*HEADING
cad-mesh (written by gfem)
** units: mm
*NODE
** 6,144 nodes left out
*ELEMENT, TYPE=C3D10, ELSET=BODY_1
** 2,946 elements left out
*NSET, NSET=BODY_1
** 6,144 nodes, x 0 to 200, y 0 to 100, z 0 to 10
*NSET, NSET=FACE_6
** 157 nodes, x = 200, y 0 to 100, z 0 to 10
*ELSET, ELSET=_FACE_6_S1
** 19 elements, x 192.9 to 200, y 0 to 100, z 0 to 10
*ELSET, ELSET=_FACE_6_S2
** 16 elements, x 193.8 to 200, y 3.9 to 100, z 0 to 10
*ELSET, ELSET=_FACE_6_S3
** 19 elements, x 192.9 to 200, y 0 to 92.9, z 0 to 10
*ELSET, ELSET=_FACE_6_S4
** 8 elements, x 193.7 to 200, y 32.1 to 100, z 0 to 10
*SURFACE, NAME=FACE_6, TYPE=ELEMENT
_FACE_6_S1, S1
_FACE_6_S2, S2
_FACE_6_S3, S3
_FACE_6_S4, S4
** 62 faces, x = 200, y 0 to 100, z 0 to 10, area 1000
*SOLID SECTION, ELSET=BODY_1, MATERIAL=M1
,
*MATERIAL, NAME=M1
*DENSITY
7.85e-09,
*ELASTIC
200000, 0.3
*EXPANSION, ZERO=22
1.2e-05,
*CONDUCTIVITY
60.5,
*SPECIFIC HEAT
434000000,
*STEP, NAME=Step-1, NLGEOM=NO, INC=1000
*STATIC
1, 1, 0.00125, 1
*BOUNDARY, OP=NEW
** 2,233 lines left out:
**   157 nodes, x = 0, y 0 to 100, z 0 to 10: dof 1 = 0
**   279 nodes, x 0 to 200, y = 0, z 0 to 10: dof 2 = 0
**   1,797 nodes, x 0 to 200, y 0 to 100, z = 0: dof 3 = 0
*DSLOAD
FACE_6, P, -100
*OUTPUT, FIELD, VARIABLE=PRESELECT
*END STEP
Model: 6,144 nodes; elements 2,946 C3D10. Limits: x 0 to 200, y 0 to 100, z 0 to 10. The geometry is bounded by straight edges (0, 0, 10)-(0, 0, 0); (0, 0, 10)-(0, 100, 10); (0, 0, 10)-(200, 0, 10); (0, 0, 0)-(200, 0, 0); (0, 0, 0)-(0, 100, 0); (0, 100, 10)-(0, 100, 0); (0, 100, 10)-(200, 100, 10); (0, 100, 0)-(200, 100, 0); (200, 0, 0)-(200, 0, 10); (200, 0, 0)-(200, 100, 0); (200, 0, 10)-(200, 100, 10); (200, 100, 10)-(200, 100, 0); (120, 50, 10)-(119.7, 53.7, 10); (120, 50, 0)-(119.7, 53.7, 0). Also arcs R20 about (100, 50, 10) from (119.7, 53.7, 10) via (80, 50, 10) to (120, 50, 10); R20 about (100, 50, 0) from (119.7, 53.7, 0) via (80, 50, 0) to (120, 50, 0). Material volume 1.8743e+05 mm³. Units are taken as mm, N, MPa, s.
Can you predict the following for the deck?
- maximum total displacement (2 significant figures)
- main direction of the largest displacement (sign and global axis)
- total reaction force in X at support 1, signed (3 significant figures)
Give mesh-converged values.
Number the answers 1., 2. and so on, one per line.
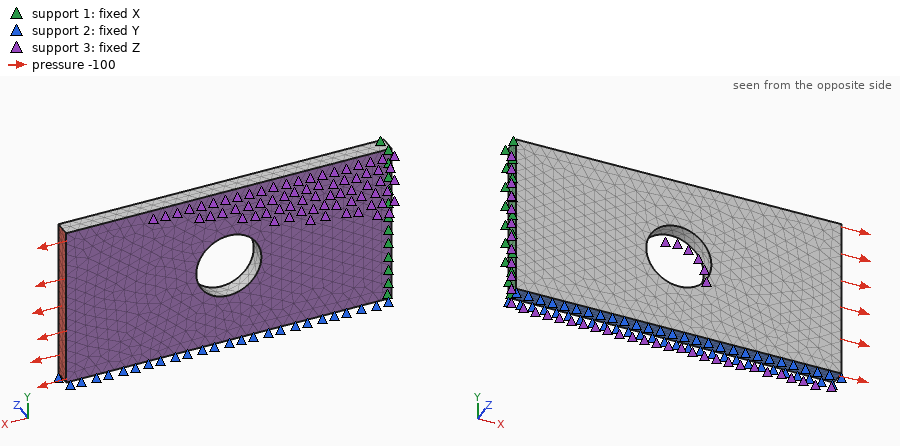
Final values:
1. 0.12 mm
2. +X
3. -100000 N
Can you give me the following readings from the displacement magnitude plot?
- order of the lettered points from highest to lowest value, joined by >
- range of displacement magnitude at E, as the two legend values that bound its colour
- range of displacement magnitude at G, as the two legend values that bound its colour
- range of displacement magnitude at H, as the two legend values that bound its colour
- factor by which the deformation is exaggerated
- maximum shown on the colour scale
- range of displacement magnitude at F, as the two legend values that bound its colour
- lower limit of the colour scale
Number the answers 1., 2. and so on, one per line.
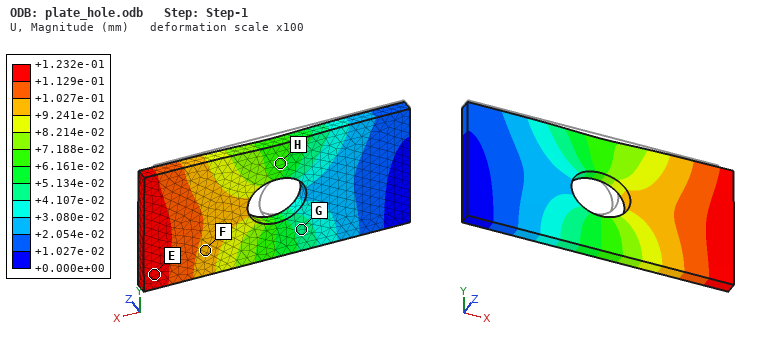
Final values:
1. E > F > H > G
2. +1.129e-01 to +1.232e-01 mm
3. +4.107e-02 to +5.134e-02 mm
4. +6.161e-02 to +7.188e-02 mm
5. 100
6. +1.232e-01 mm
7. +9.241e-02 to +1.027e-01 mm
8. +0.000e+00 mm
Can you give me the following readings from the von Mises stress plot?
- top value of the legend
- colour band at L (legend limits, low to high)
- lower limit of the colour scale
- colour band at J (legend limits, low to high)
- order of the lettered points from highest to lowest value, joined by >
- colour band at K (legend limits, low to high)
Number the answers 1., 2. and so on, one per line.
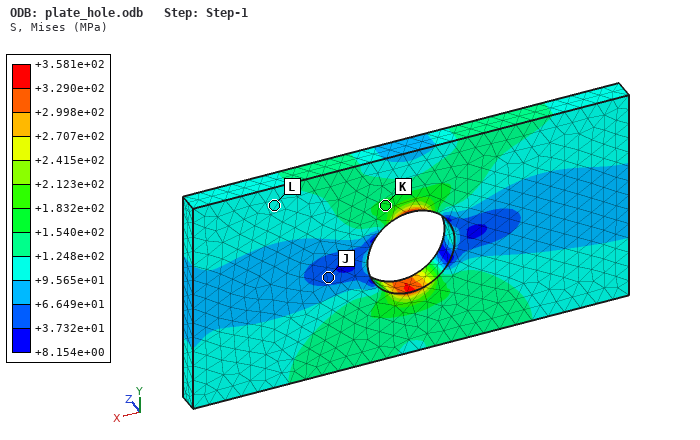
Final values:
1. +3.581e+02 MPa
2. +9.565e+01 to +1.248e+02 MPa
3. +8.154e+00 MPa
4. +3.732e+01 to +6.649e+01 MPa
5. K > L > J
6. +1.540e+02 to +1.832e+02 MPa
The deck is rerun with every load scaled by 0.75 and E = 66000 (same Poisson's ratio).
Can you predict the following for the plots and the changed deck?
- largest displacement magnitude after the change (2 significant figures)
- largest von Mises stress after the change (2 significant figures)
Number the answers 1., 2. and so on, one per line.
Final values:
1. 0.28 mm
2. 270 MPa
